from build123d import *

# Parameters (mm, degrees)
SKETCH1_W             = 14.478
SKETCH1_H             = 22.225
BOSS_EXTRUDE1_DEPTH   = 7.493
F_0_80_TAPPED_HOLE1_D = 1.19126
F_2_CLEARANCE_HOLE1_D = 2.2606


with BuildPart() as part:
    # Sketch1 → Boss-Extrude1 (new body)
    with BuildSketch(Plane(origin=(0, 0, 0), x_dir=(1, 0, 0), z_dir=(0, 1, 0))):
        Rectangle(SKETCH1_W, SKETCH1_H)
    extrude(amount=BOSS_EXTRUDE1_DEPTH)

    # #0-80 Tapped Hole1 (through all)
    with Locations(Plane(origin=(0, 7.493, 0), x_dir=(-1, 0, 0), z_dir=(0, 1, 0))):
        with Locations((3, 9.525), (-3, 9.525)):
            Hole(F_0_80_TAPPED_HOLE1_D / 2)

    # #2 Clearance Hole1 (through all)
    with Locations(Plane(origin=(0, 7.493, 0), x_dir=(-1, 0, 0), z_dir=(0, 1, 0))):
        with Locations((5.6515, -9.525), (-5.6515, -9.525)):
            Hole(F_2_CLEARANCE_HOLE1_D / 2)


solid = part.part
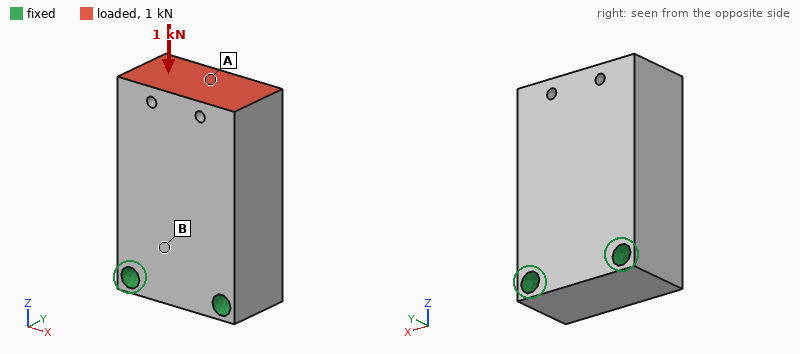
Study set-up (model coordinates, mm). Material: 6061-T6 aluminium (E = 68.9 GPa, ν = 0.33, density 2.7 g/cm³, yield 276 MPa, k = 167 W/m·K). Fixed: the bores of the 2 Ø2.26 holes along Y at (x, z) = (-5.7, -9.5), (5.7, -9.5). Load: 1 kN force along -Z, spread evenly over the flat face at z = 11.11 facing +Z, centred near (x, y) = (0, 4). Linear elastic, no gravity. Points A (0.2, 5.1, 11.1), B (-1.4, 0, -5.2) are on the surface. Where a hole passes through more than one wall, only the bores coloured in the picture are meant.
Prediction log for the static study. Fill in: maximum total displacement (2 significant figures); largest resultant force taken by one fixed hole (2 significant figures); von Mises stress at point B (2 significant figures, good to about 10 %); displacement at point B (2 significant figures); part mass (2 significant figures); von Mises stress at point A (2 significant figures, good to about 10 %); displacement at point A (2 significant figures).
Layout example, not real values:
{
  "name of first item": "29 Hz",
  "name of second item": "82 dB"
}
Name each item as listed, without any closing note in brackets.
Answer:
{
  "maximum total displacement": "3.2 µm",
  "largest resultant force taken by one fixed hole": "520 N",
  "von Mises stress at point B": "5.7 MPa",
  "displacement at point B": "0.96 µm",
  "part mass": "6.3 g",
  "von Mises stress at point A": "11 MPa",
  "displacement at point A": "3.0 µm"
}
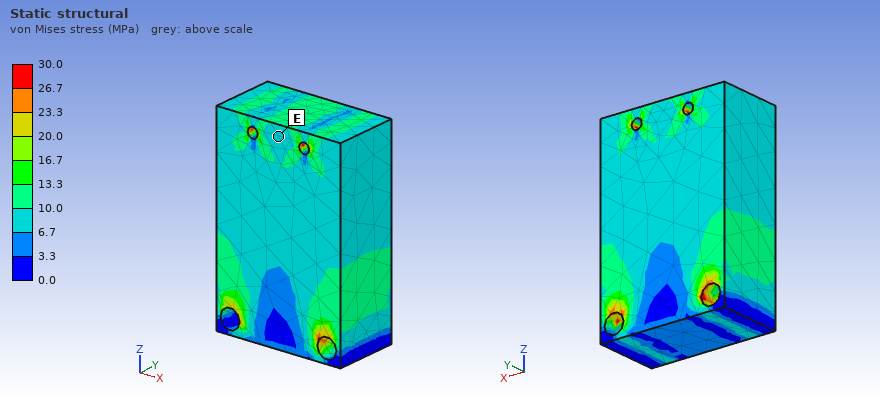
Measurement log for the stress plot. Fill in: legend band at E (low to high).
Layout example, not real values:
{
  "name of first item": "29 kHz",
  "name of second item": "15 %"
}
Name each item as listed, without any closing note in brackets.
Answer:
{
  "legend band at E": "6.7 to 10.0 MPa"
}
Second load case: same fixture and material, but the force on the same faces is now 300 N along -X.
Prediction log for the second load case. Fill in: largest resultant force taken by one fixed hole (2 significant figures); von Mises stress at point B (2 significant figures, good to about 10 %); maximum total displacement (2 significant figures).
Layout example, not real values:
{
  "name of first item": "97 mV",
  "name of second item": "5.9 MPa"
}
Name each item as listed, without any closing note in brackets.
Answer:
{
  "largest resultant force taken by one fixed hole": "540 N",
  "von Mises stress at point B": "6.0 MPa",
  "maximum total displacement": "9.6 µm"
}
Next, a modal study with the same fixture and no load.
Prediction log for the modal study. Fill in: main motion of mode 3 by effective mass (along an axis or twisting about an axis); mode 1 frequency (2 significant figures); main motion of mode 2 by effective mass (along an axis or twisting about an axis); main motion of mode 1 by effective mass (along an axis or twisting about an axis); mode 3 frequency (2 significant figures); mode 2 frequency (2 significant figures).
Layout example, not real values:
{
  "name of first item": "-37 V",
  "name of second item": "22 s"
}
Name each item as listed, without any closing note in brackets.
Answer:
{
  "main motion of mode 3 by effective mass": "twisting about Z",
  "mode 1 frequency": "12 kHz",
  "main motion of mode 2 by effective mass": "along X",
  "main motion of mode 1 by effective mass": "along Y",
  "mode 3 frequency": "31 kHz",
  "mode 2 frequency": "22 kHz"
}
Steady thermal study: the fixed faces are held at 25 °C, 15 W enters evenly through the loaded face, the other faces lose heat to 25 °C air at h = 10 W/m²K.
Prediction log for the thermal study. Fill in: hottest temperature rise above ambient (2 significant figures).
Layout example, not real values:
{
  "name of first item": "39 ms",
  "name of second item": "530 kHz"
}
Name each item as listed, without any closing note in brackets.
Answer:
{
  "hottest temperature rise above ambient": "18 K"
}
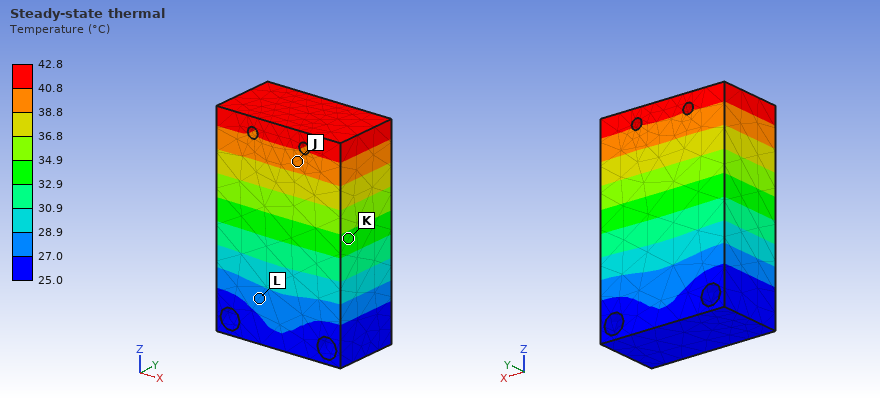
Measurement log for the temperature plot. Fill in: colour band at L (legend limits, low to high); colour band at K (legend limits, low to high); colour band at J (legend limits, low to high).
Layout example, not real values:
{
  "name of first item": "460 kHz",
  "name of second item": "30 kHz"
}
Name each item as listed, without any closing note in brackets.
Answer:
{
  "colour band at L": "27.0 to 28.9 °C",
  "colour band at K": "32.9 to 34.9 °C",
  "colour band at J": "38.8 to 40.8 °C"
}
